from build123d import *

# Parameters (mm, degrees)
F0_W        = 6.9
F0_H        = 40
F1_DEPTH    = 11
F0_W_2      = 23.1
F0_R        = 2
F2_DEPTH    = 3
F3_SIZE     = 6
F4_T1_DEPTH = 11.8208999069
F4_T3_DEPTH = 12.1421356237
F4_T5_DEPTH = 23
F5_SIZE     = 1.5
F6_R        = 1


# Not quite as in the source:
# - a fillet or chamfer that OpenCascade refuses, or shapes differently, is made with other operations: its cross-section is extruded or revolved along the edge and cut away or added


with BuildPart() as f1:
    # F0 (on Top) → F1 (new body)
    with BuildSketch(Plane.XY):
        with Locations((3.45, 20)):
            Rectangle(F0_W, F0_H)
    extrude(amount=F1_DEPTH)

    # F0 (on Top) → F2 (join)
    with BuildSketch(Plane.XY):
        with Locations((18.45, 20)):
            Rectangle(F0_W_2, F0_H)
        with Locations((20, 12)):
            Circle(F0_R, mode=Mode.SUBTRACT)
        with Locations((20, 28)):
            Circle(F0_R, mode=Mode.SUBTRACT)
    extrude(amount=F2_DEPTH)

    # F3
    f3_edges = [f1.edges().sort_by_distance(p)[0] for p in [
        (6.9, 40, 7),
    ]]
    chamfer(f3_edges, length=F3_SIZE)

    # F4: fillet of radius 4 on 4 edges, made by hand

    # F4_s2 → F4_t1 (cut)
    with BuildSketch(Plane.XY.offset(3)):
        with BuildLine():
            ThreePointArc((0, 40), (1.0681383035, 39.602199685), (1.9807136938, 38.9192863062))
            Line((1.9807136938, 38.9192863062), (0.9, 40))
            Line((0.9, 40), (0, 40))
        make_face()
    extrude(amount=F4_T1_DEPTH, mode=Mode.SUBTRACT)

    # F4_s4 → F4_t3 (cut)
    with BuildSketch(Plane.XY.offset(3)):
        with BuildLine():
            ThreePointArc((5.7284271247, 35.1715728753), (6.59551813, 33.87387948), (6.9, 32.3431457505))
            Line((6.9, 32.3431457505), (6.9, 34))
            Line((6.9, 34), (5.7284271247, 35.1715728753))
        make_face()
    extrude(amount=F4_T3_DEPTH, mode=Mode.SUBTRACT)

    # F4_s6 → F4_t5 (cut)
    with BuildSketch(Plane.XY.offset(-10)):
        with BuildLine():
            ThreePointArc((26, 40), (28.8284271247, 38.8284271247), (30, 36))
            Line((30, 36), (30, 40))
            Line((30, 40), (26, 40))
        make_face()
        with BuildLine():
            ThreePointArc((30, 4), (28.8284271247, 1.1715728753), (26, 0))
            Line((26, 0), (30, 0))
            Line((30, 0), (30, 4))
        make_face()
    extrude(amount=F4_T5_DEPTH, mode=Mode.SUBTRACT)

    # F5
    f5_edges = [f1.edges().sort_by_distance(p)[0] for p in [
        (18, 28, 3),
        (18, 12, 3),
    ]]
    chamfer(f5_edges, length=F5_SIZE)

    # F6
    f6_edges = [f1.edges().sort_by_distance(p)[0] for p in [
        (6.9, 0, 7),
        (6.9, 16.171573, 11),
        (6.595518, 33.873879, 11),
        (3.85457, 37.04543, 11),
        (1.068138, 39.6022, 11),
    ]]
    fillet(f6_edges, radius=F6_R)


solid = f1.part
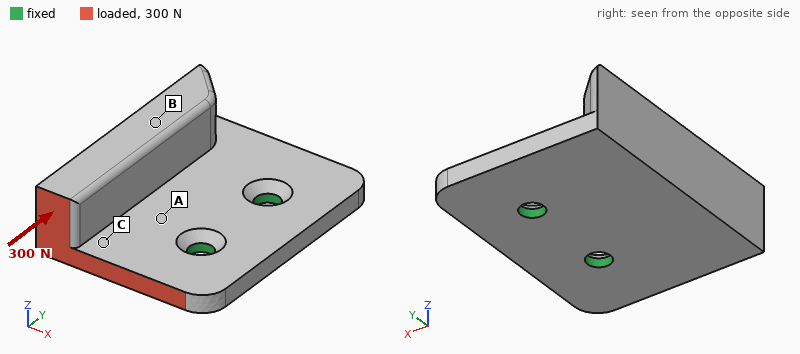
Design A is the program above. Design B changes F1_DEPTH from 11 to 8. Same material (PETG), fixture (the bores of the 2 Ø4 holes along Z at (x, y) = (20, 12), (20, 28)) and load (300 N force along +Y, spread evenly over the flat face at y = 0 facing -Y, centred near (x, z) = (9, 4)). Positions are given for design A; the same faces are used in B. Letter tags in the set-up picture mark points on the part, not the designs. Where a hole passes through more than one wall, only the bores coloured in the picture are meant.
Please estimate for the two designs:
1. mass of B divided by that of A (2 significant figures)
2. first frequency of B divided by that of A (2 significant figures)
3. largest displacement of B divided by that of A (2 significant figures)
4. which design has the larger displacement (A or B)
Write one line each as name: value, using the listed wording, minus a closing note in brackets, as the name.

mass of B divided by that of A: 0.86
first frequency of B divided by that of A: 1.2
largest displacement of B divided by that of A: 0.63
which design has the larger displacement: A
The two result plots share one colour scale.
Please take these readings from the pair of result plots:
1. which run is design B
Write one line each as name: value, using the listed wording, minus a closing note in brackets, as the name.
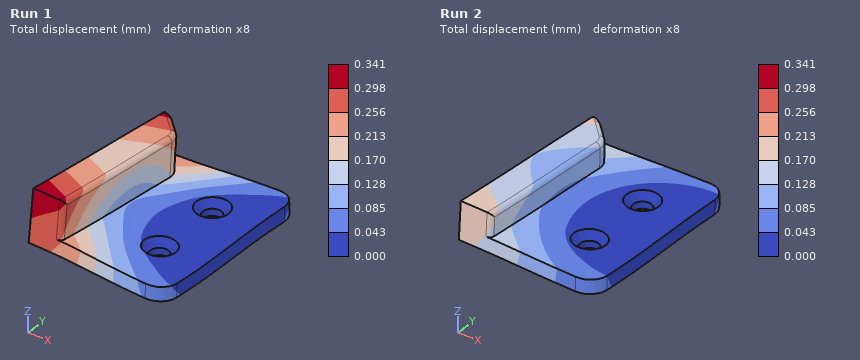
which run is design B: Run 2
